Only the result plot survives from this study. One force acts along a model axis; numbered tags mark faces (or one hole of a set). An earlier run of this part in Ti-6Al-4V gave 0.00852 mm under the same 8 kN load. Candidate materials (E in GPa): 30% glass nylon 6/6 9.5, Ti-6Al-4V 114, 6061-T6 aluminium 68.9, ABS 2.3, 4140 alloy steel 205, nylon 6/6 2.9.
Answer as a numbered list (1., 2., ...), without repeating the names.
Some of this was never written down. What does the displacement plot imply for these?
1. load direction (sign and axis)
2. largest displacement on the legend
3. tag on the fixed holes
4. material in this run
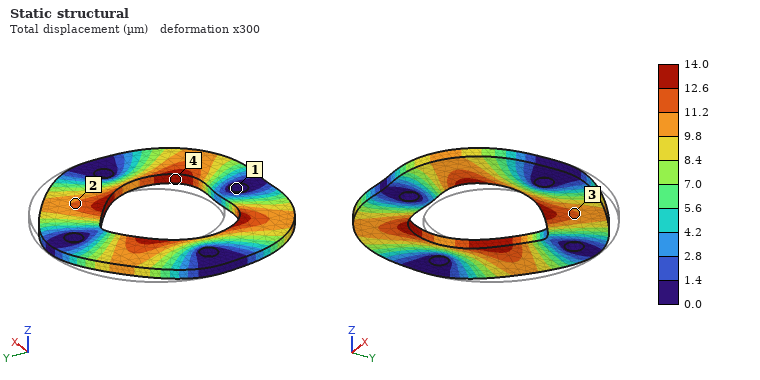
1. -Y
2. 14.0 µm
3. 1
4. 6061-T6 aluminium
